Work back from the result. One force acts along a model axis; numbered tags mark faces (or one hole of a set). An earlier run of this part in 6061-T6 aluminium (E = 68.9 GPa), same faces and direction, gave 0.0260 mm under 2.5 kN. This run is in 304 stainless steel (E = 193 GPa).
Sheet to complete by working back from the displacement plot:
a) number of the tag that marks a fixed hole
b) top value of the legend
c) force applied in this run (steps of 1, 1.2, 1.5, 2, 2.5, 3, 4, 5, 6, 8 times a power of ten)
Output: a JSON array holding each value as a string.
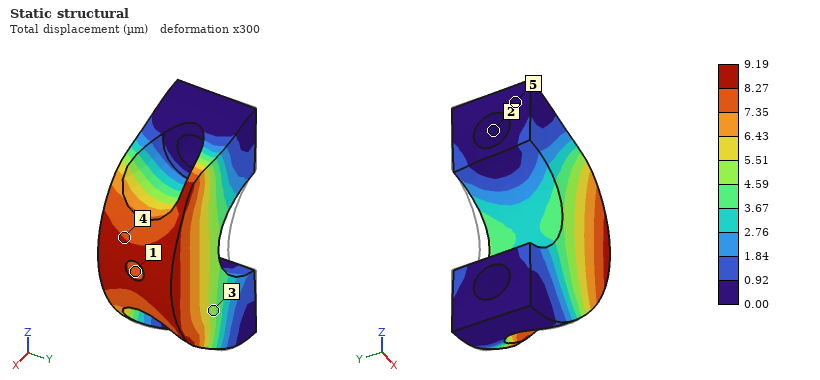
["2", "9.19 µm", "2.5 kN"]
